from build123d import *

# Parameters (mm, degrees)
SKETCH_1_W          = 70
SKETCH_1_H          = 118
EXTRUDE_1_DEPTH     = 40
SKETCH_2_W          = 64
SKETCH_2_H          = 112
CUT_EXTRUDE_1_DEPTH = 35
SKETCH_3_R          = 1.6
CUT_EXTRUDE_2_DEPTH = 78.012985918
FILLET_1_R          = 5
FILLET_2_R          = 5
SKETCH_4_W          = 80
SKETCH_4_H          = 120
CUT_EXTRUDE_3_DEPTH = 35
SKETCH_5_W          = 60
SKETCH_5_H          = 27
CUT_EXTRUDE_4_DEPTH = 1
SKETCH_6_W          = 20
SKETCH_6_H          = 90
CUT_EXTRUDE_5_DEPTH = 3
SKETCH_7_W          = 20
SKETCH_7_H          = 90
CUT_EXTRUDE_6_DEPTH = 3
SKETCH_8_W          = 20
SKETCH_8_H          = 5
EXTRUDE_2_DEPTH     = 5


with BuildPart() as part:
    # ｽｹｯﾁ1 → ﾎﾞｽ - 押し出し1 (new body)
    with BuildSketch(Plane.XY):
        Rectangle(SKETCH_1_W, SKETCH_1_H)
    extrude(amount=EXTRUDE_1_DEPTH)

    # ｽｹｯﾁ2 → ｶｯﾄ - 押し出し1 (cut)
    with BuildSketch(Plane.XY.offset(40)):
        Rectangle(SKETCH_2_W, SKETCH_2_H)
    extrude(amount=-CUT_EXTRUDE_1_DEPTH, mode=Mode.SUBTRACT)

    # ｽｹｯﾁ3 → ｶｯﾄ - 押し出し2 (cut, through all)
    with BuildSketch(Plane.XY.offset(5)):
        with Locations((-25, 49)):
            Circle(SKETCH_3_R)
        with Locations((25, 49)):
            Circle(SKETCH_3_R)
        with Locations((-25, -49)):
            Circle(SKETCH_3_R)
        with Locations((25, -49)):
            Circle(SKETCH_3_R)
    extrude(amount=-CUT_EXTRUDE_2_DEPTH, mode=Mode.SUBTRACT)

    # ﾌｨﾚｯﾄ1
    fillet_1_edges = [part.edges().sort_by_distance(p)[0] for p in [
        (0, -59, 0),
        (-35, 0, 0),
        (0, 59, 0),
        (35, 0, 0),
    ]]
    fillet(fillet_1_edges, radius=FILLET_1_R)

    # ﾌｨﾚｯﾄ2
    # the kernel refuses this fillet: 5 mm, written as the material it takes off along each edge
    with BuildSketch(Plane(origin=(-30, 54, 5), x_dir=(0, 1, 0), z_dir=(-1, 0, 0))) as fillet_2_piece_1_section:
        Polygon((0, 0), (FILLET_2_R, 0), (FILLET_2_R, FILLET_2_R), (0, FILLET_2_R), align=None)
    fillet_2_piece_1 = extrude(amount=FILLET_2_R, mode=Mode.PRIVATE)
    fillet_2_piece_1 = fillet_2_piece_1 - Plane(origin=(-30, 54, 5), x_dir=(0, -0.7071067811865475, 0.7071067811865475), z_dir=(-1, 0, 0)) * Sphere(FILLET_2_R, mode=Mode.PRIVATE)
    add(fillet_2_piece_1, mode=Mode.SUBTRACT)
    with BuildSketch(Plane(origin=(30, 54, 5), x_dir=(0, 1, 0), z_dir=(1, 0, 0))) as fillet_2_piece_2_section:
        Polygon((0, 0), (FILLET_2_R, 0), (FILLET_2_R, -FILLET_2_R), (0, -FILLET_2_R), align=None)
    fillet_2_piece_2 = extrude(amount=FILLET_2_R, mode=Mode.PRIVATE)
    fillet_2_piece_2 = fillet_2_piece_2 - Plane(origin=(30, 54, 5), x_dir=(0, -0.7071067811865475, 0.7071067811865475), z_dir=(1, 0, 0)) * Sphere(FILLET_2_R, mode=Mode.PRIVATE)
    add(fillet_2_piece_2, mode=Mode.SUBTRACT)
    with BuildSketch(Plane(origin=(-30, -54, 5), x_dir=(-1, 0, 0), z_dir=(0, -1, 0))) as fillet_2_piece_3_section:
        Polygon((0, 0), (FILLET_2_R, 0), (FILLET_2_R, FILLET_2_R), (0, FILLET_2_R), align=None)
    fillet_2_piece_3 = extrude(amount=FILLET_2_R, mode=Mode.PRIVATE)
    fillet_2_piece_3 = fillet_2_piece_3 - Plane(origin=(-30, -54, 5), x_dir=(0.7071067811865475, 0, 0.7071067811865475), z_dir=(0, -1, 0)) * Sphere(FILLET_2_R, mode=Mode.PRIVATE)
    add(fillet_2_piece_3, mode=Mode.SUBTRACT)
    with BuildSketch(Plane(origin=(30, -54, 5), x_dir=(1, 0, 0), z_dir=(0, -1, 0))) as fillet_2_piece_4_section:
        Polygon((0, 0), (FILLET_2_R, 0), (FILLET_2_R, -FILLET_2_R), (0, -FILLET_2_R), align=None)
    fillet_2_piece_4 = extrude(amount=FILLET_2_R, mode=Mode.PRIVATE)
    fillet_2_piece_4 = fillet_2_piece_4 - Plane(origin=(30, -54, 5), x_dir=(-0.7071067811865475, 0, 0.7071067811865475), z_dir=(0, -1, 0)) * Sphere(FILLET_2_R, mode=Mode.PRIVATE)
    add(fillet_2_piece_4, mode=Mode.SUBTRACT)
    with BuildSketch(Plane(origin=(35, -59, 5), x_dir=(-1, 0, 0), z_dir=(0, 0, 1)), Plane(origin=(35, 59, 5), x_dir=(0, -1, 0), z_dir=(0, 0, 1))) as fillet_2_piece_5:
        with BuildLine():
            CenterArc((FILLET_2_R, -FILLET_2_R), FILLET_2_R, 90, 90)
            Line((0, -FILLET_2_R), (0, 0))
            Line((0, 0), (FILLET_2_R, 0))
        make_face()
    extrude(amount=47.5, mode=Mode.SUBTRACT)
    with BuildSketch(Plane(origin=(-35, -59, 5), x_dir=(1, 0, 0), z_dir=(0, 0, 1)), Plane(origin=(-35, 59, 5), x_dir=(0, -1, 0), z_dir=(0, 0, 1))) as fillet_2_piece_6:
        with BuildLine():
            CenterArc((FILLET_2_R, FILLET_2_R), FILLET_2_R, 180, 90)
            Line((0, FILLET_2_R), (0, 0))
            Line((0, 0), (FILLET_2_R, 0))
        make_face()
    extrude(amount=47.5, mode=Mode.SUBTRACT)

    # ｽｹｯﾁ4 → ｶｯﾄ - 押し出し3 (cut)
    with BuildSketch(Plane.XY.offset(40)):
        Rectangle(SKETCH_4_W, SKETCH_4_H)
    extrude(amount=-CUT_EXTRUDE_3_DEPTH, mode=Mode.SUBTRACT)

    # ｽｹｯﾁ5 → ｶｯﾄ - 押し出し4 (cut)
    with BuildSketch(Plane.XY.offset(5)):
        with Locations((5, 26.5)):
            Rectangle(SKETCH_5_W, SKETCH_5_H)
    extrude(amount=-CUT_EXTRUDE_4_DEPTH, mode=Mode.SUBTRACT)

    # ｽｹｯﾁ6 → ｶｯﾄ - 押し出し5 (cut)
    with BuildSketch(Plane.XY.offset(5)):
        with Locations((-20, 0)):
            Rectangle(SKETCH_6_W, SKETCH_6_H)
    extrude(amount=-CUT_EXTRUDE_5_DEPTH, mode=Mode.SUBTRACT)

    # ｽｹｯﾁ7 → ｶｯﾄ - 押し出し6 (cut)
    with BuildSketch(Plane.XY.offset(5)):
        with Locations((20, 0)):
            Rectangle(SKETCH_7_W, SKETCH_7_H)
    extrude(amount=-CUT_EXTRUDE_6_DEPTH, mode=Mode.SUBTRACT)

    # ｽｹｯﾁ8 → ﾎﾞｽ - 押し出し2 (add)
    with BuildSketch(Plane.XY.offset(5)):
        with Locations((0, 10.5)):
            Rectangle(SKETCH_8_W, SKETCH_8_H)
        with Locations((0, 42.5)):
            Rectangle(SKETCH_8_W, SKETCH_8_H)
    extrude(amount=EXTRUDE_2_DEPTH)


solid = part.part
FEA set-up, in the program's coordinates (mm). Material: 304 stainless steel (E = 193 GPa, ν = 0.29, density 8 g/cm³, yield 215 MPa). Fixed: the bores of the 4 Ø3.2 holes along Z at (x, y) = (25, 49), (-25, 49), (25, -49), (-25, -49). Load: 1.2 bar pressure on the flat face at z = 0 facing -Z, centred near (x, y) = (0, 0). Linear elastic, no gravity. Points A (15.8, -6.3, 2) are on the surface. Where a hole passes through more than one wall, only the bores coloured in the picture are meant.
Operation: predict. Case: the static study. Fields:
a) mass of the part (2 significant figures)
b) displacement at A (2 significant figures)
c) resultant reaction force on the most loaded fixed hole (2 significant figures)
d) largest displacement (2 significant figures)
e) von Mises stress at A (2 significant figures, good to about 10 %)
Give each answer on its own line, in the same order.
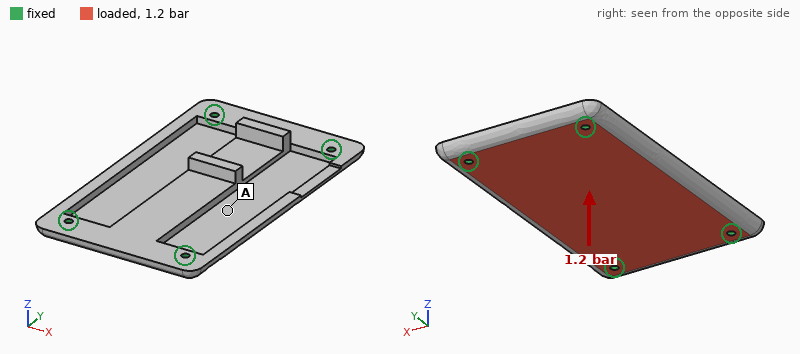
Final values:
230 g
37 µm
200 N
39 µm
9.8 MPa
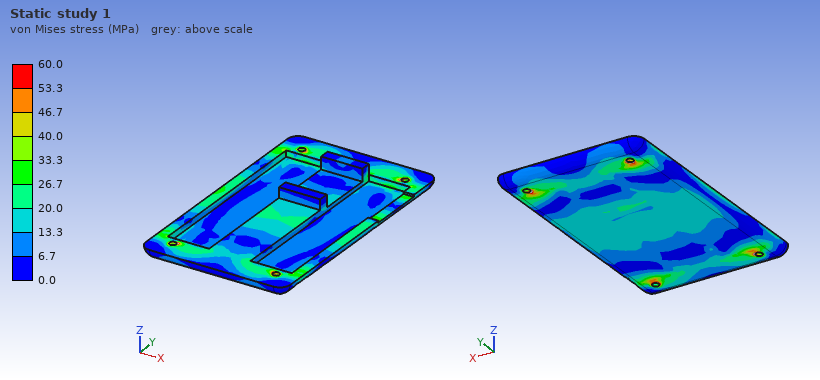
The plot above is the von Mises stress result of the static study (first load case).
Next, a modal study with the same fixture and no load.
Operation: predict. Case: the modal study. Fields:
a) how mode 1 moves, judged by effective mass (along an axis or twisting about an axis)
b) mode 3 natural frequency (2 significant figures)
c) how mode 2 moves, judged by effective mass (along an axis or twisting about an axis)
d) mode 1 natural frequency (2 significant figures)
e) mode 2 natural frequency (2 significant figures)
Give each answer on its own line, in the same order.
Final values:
along Z
4000 Hz
twisting about Y
1900 Hz
2800 Hz
